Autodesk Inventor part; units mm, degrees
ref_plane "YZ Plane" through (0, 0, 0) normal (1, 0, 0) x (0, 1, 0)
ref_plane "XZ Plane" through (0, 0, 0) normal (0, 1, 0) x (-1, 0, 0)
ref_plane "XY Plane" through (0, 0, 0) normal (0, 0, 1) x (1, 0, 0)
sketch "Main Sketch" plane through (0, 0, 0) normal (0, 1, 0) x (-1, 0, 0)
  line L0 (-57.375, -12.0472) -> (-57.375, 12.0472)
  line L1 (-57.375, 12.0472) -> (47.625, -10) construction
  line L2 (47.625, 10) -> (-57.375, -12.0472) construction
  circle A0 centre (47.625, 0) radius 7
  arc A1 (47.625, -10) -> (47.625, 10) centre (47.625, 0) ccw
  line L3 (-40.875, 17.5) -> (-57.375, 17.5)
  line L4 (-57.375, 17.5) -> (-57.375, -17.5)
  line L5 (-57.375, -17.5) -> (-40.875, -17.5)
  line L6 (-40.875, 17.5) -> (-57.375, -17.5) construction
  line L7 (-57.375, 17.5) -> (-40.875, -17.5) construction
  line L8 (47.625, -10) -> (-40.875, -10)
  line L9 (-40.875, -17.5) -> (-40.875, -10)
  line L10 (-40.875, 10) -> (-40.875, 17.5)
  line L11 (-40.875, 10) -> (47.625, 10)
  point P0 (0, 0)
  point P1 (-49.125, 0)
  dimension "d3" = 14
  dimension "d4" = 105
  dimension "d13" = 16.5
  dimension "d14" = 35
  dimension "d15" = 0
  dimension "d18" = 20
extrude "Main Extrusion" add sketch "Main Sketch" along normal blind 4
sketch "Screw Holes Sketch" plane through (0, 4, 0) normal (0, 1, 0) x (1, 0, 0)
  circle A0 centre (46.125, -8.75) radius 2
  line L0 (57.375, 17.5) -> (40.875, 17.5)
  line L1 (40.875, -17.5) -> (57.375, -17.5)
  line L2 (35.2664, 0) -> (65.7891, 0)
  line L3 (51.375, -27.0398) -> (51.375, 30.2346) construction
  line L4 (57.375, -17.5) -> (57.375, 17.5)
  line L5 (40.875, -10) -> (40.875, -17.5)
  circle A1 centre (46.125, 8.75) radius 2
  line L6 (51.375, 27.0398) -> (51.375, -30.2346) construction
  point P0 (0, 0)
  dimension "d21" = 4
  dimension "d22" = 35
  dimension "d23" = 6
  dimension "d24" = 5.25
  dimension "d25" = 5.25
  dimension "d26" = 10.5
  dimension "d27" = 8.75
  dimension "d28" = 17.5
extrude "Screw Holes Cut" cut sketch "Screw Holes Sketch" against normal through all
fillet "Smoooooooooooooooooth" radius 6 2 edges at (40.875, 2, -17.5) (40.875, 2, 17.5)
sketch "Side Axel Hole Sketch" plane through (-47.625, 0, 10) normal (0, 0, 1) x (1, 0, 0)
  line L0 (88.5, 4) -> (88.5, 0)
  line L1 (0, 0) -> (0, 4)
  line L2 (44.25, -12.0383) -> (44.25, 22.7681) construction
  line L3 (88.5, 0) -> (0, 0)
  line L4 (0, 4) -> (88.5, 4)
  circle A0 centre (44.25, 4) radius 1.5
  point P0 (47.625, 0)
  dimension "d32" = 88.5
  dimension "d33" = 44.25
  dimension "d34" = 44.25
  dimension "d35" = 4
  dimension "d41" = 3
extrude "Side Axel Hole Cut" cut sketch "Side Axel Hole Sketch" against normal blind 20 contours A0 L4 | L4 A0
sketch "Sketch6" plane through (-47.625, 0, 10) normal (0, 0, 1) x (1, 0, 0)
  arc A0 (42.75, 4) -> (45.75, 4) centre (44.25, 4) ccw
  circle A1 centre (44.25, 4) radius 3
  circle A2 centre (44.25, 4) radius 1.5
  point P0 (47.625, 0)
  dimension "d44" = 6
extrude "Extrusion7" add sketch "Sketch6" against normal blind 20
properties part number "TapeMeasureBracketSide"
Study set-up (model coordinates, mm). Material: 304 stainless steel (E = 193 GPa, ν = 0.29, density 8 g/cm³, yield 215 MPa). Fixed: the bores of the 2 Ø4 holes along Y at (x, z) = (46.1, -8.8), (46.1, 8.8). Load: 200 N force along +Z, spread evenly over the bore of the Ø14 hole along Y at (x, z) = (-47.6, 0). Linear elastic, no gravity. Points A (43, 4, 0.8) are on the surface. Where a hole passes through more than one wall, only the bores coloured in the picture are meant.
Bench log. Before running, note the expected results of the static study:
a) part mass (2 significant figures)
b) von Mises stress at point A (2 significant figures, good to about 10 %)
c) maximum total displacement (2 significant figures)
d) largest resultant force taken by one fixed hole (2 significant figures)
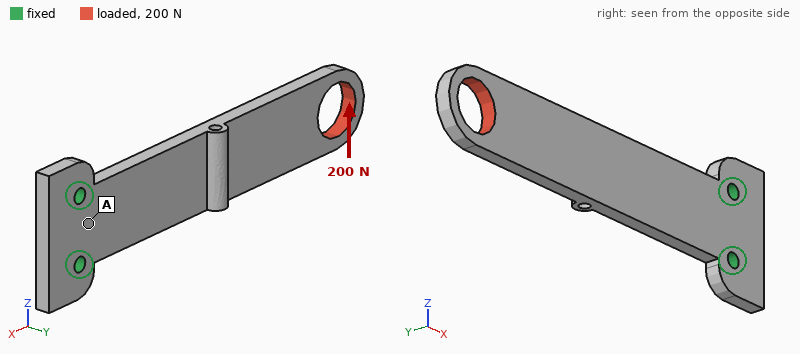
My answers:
75 g
9.4 MPa
0.13 mm
1.1 kN
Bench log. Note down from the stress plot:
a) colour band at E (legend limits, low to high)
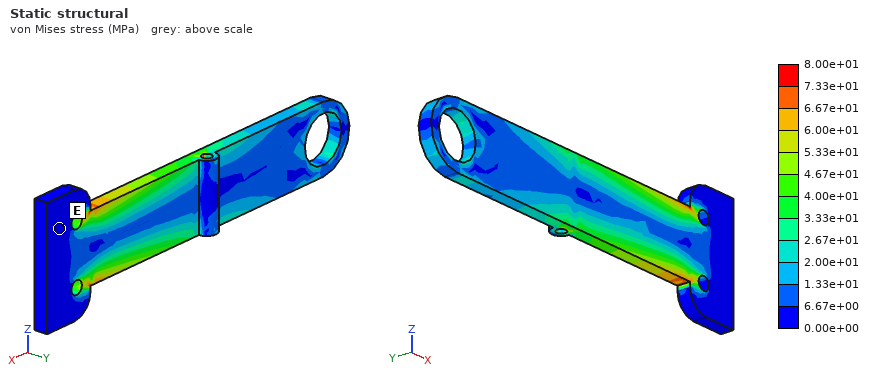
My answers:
0.00e+00 to 6.67e+00 MPa
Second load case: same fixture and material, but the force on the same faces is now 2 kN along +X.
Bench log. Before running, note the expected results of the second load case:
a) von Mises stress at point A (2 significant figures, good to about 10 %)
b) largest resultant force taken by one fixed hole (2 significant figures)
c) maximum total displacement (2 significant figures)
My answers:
12 MPa
1.0 kN
24 µm
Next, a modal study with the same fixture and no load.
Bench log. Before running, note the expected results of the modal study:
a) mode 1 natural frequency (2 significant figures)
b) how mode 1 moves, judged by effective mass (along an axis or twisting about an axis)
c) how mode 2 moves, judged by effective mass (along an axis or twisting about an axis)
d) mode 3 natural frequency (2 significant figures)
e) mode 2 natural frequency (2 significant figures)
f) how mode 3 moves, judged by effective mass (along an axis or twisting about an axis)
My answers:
360 Hz
along Y
along Z
2100 Hz
1800 Hz
along Y
